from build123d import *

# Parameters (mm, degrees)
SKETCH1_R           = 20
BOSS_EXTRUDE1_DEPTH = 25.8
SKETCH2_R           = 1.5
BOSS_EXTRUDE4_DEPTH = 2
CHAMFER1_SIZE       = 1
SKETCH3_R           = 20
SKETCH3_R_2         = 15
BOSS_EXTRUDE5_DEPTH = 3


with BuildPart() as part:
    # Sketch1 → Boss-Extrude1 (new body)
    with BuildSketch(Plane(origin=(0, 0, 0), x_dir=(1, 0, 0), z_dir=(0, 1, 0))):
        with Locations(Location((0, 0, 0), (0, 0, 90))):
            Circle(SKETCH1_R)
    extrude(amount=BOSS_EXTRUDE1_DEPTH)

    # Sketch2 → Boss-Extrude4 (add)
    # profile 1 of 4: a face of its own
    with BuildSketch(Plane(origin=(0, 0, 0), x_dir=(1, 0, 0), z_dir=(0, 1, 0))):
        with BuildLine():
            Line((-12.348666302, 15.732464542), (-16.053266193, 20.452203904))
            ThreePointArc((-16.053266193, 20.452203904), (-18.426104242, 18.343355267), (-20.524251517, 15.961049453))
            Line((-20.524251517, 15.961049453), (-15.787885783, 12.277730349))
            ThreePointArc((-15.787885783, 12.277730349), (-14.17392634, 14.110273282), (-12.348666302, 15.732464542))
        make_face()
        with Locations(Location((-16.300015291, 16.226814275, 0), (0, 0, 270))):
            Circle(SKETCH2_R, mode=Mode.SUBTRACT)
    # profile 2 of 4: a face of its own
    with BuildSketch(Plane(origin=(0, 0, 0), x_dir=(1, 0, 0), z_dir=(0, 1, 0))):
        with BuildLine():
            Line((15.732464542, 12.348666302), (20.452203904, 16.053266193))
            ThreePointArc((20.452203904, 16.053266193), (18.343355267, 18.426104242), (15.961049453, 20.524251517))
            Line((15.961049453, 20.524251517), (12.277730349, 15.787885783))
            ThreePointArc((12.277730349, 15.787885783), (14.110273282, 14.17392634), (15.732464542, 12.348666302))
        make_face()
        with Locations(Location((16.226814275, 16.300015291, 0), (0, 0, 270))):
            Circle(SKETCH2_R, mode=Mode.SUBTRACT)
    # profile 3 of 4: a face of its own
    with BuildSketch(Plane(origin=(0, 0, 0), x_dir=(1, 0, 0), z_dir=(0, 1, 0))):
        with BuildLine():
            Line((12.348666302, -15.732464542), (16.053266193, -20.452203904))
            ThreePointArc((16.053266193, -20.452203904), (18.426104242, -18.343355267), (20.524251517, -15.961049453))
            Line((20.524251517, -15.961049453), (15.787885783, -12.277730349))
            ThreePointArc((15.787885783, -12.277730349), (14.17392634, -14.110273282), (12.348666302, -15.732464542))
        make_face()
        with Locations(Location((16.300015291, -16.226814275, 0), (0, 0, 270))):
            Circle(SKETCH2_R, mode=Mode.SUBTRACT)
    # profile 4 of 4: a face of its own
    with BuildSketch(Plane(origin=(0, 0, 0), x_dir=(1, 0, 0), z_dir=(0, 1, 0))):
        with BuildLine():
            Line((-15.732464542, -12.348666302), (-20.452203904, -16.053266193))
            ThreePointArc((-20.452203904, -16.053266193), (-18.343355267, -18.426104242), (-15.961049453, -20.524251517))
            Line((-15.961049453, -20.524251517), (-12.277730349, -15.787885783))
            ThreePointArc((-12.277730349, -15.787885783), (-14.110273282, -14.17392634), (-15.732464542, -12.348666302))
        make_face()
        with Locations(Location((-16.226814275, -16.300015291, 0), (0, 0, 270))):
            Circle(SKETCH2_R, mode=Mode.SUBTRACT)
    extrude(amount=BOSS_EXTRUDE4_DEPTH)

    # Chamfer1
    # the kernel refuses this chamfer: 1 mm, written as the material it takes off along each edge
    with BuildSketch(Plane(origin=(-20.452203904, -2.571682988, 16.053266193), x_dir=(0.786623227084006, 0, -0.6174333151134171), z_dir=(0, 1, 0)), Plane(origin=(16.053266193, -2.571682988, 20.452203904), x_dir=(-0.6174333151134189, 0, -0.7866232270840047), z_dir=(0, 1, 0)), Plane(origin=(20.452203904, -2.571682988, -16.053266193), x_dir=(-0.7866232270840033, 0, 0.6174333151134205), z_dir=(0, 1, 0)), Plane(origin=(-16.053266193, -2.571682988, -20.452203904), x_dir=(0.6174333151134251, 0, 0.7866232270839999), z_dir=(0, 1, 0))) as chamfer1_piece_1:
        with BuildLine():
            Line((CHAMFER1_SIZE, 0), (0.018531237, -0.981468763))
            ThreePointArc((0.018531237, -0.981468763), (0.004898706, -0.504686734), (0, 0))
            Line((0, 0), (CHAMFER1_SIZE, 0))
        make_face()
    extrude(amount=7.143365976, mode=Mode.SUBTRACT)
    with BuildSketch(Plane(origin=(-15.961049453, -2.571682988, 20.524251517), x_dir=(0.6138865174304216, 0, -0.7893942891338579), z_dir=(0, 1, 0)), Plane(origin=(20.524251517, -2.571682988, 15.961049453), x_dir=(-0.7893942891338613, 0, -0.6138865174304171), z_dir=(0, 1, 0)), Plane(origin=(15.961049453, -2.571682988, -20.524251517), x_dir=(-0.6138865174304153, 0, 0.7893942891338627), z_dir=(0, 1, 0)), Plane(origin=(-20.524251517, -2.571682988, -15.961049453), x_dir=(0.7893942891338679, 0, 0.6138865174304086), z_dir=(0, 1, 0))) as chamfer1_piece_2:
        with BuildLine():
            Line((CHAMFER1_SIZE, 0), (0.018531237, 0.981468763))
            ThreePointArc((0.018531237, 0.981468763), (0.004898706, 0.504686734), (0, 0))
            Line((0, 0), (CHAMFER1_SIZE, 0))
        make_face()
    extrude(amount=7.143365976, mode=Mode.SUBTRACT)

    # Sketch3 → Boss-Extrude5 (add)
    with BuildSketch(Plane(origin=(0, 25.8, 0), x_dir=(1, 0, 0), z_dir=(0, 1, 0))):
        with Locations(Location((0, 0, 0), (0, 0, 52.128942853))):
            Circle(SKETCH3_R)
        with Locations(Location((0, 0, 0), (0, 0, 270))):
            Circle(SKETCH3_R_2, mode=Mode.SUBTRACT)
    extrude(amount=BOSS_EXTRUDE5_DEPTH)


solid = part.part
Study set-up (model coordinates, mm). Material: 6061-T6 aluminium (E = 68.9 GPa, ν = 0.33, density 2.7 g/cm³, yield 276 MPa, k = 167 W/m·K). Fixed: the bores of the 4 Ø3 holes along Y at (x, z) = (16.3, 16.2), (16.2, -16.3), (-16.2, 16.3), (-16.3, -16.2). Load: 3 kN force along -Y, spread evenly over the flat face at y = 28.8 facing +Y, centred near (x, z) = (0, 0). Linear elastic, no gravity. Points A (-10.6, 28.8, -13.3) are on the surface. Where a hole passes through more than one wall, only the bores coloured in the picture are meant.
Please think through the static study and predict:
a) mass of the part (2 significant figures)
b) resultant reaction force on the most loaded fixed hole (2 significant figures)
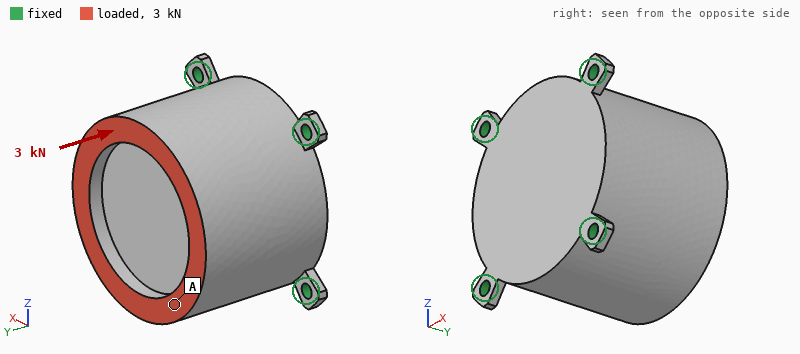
93 g
830 N
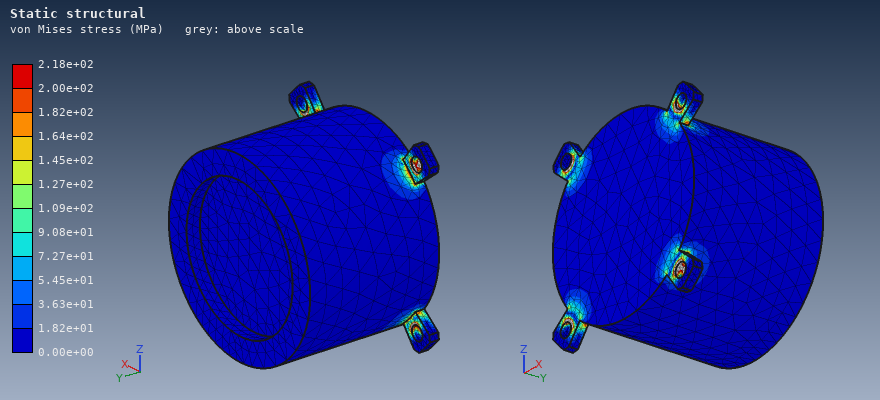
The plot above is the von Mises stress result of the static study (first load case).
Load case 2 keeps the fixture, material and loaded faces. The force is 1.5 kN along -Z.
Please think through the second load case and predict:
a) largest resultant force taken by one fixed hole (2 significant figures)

860 N
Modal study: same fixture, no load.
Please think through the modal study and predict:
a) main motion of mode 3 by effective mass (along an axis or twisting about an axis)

along Y
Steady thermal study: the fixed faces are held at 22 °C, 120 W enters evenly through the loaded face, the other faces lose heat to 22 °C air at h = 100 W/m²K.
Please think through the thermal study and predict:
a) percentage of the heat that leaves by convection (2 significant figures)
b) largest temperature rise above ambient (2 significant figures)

26 %
67 K
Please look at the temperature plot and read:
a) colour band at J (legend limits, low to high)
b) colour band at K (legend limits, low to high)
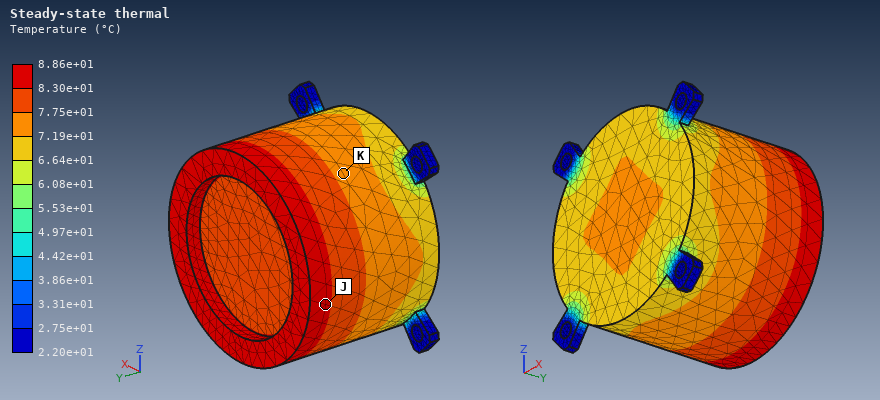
8.30e+01 to 8.86e+01 °C
7.19e+01 to 7.75e+01 °C
